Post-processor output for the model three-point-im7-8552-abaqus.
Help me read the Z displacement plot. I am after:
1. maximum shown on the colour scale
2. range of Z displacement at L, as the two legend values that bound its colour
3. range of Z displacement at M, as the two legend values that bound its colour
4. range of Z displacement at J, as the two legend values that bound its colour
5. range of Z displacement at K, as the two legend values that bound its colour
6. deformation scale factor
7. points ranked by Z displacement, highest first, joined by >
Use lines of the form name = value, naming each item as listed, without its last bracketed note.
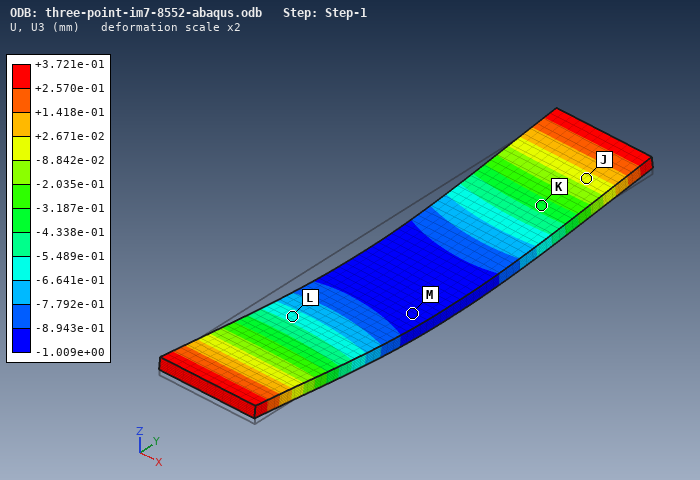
maximum shown on the colour scale = +3.721e-01 mm
range of Z displacement at L, as the two legend values that bound its colour = -6.641e-01 to -5.489e-01 mm
range of Z displacement at M, as the two legend values that bound its colour = -1.009e+00 to -8.943e-01 mm
range of Z displacement at J, as the two legend values that bound its colour = -8.842e-02 to +2.671e-02 mm
range of Z displacement at K, as the two legend values that bound its colour = -4.338e-01 to -3.187e-01 mm
deformation scale factor = 2
points ranked by Z displacement, highest first, joined by > = J > K > L > M
